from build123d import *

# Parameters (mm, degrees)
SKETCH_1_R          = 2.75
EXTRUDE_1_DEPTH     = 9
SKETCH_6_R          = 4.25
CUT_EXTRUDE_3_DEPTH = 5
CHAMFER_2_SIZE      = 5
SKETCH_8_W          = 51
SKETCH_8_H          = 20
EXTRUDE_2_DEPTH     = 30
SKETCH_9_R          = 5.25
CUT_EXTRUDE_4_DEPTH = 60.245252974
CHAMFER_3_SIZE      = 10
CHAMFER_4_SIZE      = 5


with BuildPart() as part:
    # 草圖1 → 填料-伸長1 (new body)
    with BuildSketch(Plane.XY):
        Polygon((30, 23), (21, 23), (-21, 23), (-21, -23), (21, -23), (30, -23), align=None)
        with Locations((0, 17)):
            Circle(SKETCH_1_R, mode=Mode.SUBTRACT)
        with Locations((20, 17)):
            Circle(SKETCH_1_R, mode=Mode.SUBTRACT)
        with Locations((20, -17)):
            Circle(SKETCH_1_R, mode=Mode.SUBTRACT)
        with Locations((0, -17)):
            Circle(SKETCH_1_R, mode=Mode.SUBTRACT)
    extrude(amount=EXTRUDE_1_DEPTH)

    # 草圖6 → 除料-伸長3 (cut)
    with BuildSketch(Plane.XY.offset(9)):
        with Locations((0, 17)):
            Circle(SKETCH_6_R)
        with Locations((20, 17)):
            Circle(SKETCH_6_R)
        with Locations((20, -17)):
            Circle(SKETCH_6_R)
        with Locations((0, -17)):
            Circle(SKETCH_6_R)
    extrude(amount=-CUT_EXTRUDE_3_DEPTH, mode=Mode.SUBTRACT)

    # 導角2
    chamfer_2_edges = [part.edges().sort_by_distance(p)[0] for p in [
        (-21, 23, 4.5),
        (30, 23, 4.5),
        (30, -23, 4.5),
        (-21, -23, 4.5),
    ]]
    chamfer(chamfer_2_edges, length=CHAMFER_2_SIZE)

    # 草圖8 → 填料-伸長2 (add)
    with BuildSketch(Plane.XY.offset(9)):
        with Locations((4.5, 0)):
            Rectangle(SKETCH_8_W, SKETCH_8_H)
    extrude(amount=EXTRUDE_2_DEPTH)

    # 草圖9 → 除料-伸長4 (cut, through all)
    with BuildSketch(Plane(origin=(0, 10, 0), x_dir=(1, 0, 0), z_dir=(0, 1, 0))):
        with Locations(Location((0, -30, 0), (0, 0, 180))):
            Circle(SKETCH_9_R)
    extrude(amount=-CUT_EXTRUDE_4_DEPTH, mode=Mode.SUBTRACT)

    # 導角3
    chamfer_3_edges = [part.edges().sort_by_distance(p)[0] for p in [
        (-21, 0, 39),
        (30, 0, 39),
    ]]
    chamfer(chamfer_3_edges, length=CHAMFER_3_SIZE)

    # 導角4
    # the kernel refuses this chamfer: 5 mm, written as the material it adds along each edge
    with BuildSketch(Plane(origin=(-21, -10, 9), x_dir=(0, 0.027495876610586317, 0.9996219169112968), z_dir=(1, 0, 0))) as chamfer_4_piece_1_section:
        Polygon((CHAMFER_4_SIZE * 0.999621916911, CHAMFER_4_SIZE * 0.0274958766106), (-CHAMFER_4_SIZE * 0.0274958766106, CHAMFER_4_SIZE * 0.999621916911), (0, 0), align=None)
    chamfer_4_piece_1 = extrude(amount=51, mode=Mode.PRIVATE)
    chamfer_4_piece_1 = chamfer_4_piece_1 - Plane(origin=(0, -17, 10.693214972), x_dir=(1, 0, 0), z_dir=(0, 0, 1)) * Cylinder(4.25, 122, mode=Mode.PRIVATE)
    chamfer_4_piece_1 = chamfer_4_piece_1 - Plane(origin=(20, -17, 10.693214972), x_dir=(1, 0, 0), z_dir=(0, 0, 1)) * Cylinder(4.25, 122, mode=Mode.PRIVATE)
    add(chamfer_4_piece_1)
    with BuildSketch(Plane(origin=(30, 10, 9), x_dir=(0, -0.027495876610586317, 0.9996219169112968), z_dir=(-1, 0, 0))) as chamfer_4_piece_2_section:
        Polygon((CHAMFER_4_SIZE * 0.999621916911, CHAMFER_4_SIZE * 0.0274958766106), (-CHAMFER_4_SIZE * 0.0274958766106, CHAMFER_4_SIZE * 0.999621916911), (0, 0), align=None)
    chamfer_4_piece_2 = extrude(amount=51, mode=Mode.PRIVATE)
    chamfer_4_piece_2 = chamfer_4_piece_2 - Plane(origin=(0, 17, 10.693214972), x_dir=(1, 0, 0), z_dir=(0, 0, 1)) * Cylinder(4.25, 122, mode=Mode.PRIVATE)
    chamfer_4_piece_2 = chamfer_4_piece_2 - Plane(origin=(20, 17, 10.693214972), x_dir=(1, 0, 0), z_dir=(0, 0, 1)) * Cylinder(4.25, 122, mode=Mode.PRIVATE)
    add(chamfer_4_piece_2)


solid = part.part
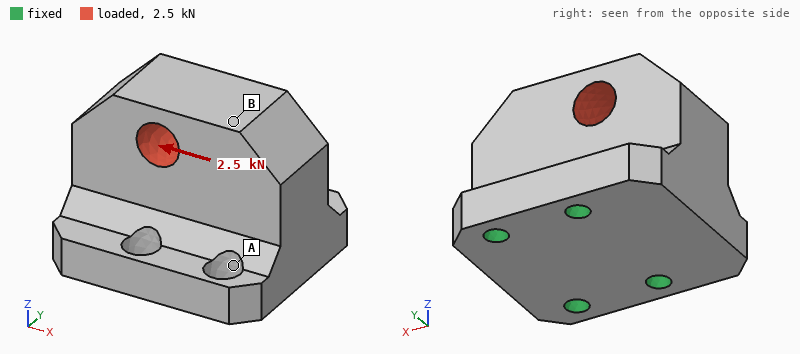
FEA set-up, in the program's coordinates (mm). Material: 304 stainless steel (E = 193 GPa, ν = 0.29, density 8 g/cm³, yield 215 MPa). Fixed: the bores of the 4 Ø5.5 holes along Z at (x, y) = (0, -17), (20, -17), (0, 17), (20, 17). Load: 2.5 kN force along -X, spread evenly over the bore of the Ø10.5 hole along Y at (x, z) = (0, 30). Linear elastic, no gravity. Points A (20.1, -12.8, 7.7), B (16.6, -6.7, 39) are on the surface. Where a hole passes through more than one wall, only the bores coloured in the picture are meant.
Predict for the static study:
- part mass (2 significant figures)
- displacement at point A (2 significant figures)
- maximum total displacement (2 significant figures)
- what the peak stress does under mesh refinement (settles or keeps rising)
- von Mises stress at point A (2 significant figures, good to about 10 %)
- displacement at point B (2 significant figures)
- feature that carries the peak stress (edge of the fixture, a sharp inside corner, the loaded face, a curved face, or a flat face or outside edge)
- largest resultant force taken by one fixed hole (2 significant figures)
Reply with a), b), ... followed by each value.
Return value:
a) 380 g
b) 2.1 µm
c) 11 µm
d) keeps rising
e) 20 MPa
f) 9.4 µm
g) edge of the fixture
h) 1.8 kN
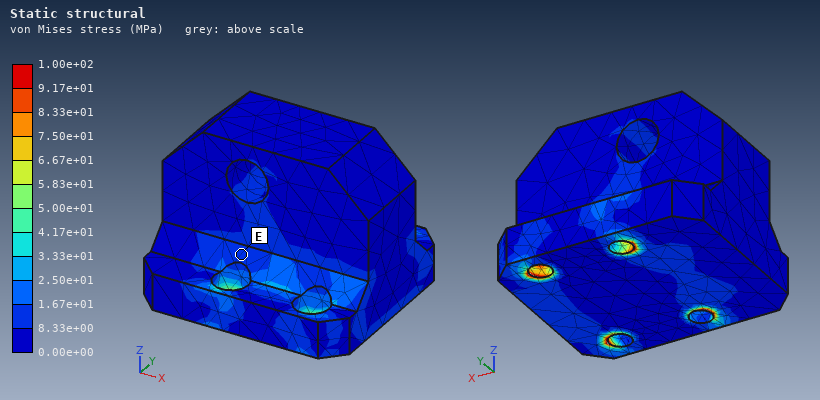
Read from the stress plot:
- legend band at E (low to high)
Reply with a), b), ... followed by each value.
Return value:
a) 8.33e+00 to 1.67e+01 MPa
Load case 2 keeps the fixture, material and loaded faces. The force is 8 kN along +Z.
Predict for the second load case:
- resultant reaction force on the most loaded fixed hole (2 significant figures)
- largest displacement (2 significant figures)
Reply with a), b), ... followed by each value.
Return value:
a) 4.0 kN
b) 13 µm
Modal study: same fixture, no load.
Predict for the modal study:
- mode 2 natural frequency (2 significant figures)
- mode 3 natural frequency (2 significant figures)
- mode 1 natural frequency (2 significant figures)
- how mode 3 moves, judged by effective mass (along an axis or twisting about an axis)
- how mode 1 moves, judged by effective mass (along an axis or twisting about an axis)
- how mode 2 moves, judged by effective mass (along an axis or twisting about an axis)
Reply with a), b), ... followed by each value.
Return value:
a) 10 kHz
b) 14 kHz
c) 6300 Hz
d) along Z
e) along X
f) along Y
